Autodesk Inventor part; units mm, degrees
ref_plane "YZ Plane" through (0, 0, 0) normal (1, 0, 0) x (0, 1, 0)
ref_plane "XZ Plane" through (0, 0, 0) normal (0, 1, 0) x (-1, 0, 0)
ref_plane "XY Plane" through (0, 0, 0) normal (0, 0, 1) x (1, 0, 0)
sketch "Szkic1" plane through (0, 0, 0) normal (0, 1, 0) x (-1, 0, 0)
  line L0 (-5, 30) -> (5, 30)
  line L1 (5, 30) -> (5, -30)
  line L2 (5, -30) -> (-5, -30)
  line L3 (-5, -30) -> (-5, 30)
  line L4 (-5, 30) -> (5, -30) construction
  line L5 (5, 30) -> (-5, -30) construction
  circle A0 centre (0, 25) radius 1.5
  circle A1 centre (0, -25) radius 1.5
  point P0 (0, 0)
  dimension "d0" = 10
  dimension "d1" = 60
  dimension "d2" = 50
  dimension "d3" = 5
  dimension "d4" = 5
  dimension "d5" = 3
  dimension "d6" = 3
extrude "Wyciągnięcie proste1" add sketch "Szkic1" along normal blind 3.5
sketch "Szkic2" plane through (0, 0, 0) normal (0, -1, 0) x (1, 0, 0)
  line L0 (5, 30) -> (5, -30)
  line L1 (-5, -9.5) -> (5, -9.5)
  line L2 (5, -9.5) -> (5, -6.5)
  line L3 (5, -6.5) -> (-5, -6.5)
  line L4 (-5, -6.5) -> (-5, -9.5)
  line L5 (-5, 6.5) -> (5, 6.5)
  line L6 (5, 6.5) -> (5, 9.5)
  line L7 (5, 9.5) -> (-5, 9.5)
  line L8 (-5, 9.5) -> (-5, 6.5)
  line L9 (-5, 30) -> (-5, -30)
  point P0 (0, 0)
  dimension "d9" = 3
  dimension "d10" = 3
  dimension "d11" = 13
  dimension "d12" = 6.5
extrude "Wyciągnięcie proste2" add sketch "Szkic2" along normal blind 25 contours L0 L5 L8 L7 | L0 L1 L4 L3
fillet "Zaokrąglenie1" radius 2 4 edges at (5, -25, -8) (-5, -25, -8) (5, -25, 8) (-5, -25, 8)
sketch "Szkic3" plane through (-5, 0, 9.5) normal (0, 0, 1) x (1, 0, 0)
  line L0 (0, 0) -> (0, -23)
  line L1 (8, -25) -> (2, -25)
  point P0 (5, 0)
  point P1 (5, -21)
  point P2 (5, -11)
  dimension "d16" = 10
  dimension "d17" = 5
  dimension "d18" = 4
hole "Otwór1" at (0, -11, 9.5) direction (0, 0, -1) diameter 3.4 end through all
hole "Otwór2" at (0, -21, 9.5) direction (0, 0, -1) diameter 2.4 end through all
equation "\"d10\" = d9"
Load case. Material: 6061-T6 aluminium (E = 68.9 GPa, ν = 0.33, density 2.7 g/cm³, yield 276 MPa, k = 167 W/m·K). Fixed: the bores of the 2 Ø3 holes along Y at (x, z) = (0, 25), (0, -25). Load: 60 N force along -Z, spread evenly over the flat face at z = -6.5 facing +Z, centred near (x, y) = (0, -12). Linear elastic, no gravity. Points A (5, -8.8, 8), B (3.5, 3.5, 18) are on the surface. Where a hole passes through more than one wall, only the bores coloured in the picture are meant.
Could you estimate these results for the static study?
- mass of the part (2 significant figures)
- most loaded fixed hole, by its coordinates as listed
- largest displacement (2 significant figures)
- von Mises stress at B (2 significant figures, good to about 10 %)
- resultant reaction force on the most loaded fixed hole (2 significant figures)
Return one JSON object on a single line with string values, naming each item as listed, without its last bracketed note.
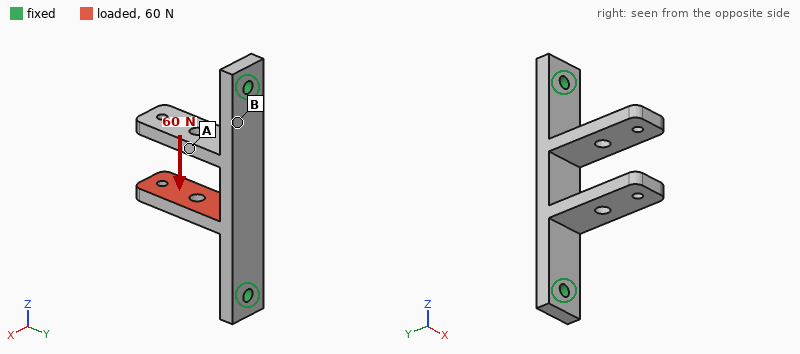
{"mass of the part": "9.3 g", "most loaded fixed hole, by its coordinates as listed": "(0, -25)", "largest displacement": "0.12 mm", "von Mises stress at B": "6.5 MPa", "resultant reaction force on the most loaded fixed hole": "44 N"}
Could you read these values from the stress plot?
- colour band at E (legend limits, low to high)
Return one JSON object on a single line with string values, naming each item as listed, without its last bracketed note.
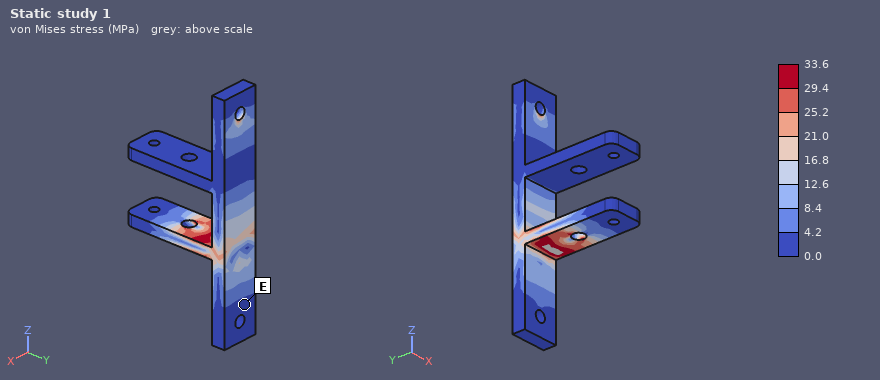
{"colour band at E": "0.0 to 4.2 MPa"}
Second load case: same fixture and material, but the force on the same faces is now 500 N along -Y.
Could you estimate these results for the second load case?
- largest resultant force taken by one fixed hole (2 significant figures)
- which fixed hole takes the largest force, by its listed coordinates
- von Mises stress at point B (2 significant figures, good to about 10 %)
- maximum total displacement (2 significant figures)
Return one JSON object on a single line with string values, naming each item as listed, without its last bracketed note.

{"largest resultant force taken by one fixed hole": "350 N", "which fixed hole takes the largest force, by its listed coordinates": "(0, -25)", "von Mises stress at point B": "52 MPa", "maximum total displacement": "0.27 mm"}
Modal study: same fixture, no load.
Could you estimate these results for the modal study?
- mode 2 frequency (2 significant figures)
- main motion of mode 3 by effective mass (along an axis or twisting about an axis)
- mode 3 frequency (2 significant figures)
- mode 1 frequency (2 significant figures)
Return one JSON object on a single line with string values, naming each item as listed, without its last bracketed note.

{"mode 2 frequency": "3000 Hz", "main motion of mode 3 by effective mass": "along Z", "mode 3 frequency": "3500 Hz", "mode 1 frequency": "2900 Hz"}
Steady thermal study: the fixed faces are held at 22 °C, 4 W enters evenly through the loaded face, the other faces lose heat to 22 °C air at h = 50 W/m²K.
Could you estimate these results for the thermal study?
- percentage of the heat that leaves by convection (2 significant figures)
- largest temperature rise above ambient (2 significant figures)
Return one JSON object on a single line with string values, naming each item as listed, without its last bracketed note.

{"percentage of the heat that leaves by convection": "15 %", "largest temperature rise above ambient": "17 K"}
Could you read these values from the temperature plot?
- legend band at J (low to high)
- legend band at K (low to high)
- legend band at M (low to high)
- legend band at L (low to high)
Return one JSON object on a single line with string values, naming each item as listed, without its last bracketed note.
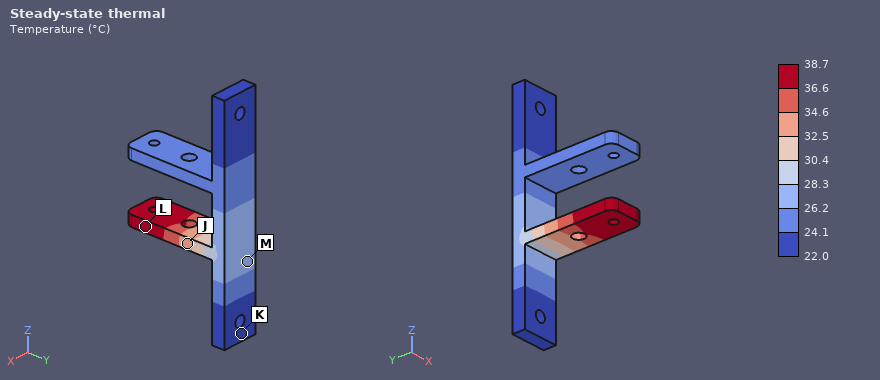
{"legend band at J": "32.5 to 34.6 °C", "legend band at K": "22.0 to 24.1 °C", "legend band at M": "26.2 to 28.3 °C", "legend band at L": "36.6 to 38.7 °C"}
